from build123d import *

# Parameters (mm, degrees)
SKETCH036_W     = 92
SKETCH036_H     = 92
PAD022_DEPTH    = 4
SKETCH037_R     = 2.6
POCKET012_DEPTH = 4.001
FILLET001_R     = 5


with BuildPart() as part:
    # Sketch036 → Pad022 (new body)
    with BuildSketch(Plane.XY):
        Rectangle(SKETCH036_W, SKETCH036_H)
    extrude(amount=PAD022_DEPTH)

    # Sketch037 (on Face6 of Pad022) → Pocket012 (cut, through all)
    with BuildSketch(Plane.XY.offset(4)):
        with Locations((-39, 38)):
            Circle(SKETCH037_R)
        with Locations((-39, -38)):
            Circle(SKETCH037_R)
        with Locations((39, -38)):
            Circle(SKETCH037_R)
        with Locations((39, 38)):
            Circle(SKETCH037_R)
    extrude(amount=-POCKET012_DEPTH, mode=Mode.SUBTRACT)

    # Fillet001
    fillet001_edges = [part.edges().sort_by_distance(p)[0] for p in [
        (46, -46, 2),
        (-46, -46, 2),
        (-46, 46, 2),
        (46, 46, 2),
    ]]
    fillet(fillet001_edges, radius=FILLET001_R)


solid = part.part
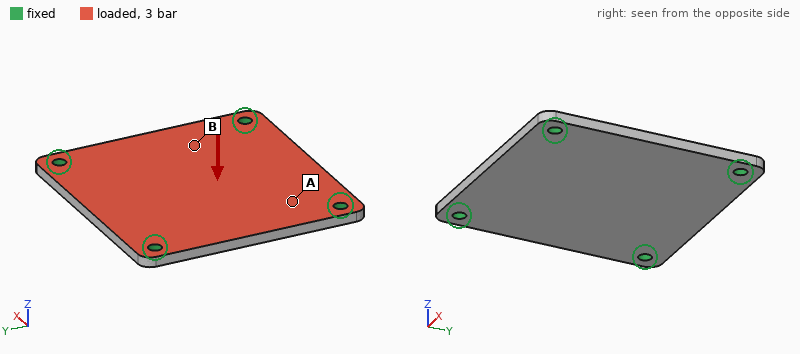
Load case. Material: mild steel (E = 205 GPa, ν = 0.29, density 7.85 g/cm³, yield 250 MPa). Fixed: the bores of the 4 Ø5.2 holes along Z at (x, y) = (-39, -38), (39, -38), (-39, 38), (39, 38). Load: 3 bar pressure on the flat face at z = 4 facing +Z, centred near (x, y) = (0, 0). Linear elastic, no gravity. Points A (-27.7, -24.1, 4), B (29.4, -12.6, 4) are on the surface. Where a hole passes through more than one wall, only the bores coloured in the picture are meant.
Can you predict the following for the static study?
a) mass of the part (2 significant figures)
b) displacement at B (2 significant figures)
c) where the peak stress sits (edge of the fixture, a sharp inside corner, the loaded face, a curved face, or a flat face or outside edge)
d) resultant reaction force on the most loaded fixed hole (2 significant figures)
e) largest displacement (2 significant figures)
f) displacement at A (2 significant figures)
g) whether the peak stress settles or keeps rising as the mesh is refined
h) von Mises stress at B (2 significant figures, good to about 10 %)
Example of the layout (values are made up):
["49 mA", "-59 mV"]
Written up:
["260 g", "38 µm", "edge of the fixture", "630 N", "65 µm", "26 µm", "keeps rising", "25 MPa"]
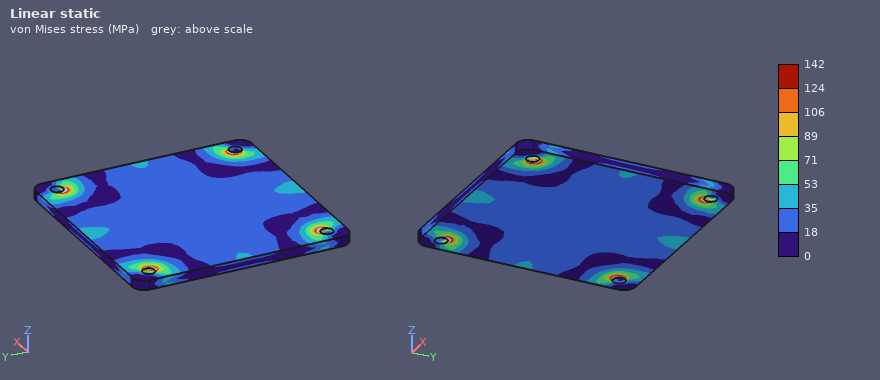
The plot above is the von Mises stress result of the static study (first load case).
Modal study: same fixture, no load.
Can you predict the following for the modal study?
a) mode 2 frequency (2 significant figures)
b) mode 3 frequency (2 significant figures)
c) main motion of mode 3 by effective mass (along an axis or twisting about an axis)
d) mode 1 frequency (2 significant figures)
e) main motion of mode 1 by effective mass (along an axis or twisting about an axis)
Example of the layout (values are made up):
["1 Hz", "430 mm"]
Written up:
["3900 Hz", "4100 Hz", "twisting about Y", "2300 Hz", "along Z"]
